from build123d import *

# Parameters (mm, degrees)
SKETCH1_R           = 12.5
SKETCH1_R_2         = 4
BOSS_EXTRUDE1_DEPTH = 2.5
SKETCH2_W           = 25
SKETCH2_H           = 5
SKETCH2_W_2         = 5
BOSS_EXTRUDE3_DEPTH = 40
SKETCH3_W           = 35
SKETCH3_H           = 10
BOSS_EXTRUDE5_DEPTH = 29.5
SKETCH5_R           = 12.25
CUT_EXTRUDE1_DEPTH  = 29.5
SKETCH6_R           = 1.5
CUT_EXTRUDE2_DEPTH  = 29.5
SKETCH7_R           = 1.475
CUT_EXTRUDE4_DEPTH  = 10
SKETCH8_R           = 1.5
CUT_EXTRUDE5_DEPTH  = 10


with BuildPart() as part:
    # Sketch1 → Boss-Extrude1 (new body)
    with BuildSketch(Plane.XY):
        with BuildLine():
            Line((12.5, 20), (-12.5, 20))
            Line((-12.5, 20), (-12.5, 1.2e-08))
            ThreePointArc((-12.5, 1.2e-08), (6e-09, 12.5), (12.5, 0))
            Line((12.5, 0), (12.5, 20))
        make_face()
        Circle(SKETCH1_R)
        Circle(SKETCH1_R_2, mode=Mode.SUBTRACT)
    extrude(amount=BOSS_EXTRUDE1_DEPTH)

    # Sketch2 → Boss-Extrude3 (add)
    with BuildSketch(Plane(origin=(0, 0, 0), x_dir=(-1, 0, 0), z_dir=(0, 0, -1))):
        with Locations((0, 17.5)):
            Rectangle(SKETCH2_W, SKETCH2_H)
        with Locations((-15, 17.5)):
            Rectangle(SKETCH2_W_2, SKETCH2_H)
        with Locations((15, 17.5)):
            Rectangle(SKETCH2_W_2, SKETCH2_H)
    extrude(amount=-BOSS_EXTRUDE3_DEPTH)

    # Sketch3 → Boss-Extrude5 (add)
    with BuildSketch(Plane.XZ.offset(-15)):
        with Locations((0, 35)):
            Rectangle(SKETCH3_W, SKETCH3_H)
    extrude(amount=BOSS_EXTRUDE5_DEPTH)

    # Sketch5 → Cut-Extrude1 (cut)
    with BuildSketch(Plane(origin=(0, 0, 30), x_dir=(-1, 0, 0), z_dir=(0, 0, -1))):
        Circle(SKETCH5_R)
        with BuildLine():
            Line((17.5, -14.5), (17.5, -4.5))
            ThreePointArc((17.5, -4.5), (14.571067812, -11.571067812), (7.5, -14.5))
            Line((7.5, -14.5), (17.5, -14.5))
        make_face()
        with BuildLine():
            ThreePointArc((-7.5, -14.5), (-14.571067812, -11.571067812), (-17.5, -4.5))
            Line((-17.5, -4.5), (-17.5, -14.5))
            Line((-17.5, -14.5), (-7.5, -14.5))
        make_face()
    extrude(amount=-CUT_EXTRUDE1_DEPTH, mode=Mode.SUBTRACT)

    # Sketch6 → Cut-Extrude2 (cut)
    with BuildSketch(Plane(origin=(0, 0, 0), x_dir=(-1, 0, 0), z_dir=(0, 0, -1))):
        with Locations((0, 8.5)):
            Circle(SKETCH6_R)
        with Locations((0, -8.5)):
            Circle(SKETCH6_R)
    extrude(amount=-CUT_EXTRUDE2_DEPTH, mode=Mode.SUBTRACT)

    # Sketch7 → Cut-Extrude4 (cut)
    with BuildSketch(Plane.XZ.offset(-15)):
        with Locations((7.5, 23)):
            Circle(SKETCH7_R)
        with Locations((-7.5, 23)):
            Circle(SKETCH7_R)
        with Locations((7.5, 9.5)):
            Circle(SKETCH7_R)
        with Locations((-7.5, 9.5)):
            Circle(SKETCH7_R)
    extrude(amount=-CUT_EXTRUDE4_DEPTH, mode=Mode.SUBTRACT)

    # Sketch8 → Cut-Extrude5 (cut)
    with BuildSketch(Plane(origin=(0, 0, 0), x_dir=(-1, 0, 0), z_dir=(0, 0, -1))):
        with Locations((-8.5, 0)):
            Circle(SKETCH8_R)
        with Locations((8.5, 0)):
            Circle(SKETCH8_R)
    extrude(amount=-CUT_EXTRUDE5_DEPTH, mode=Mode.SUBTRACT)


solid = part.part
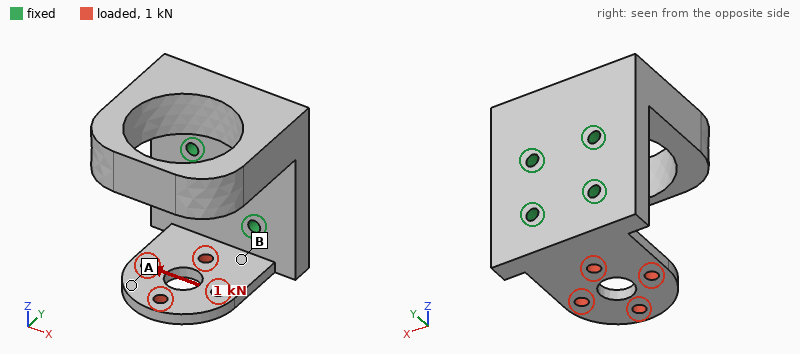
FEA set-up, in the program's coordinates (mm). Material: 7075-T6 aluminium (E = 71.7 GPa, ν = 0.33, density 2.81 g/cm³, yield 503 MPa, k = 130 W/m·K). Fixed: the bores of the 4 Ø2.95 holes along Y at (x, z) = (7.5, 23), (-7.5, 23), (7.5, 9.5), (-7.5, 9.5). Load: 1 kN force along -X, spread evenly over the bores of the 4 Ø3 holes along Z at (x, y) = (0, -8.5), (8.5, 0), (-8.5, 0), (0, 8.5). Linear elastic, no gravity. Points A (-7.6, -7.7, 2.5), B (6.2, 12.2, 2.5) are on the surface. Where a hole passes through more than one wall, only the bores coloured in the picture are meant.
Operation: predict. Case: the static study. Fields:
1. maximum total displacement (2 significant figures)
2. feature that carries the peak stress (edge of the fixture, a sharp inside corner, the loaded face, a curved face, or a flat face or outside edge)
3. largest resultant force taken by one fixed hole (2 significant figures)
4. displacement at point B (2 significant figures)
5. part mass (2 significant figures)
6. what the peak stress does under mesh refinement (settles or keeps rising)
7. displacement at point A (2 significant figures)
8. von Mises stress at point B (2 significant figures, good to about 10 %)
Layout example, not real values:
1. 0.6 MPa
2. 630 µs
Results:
1. 92 µm
2. edge of the fixture
3. 1.2 kN
4. 19 µm
5. 38 g
6. keeps rising
7. 84 µm
8. 50 MPa
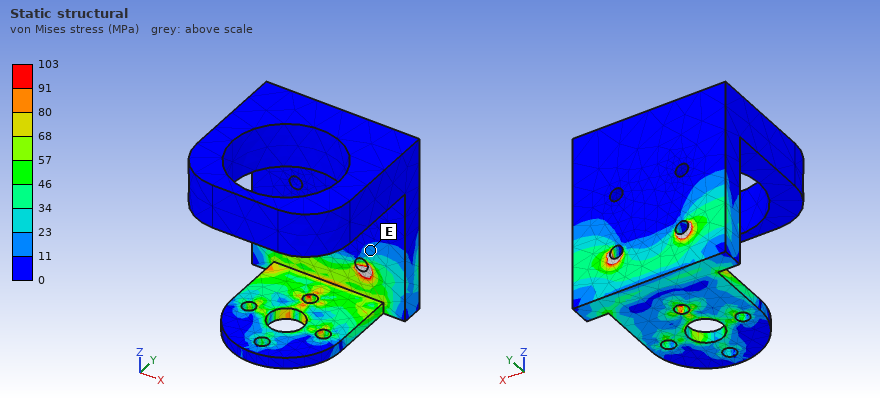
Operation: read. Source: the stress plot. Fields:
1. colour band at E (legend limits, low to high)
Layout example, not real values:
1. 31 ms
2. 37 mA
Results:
1. 11 to 23 MPa
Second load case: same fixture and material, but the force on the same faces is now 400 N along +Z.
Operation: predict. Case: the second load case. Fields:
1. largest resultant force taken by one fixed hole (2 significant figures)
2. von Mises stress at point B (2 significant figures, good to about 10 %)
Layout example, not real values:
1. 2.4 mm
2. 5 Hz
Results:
1. 210 N
2. 170 MPa
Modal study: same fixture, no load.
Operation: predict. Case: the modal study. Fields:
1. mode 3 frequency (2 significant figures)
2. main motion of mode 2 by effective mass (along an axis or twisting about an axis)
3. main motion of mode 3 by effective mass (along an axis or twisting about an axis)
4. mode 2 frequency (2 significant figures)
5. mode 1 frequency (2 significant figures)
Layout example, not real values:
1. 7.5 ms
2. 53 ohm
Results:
1. 4900 Hz
2. along Z
3. along X
4. 3000 Hz
5. 2900 Hz
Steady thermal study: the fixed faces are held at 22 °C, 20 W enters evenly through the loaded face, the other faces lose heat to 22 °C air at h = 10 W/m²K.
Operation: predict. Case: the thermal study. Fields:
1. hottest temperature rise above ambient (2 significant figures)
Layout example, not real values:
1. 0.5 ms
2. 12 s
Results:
1. 61 K
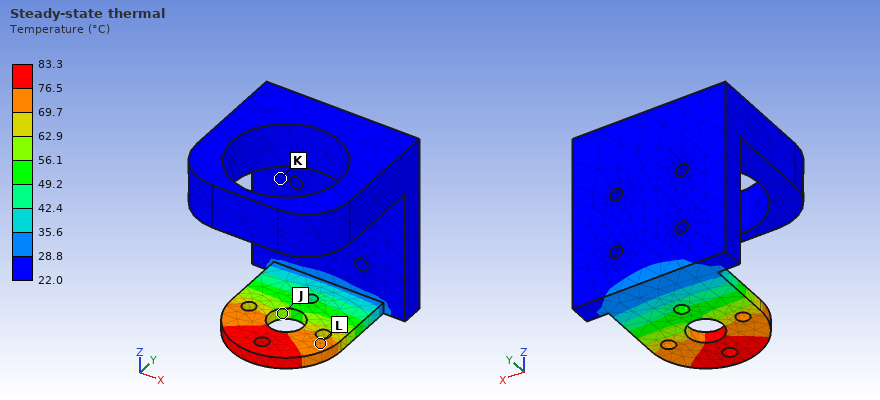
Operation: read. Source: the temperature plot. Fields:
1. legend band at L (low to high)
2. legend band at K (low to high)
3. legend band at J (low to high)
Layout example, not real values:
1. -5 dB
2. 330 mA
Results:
1. 69.7 to 76.5 °C
2. 22.0 to 28.8 °C
3. 56.1 to 62.9 °C
